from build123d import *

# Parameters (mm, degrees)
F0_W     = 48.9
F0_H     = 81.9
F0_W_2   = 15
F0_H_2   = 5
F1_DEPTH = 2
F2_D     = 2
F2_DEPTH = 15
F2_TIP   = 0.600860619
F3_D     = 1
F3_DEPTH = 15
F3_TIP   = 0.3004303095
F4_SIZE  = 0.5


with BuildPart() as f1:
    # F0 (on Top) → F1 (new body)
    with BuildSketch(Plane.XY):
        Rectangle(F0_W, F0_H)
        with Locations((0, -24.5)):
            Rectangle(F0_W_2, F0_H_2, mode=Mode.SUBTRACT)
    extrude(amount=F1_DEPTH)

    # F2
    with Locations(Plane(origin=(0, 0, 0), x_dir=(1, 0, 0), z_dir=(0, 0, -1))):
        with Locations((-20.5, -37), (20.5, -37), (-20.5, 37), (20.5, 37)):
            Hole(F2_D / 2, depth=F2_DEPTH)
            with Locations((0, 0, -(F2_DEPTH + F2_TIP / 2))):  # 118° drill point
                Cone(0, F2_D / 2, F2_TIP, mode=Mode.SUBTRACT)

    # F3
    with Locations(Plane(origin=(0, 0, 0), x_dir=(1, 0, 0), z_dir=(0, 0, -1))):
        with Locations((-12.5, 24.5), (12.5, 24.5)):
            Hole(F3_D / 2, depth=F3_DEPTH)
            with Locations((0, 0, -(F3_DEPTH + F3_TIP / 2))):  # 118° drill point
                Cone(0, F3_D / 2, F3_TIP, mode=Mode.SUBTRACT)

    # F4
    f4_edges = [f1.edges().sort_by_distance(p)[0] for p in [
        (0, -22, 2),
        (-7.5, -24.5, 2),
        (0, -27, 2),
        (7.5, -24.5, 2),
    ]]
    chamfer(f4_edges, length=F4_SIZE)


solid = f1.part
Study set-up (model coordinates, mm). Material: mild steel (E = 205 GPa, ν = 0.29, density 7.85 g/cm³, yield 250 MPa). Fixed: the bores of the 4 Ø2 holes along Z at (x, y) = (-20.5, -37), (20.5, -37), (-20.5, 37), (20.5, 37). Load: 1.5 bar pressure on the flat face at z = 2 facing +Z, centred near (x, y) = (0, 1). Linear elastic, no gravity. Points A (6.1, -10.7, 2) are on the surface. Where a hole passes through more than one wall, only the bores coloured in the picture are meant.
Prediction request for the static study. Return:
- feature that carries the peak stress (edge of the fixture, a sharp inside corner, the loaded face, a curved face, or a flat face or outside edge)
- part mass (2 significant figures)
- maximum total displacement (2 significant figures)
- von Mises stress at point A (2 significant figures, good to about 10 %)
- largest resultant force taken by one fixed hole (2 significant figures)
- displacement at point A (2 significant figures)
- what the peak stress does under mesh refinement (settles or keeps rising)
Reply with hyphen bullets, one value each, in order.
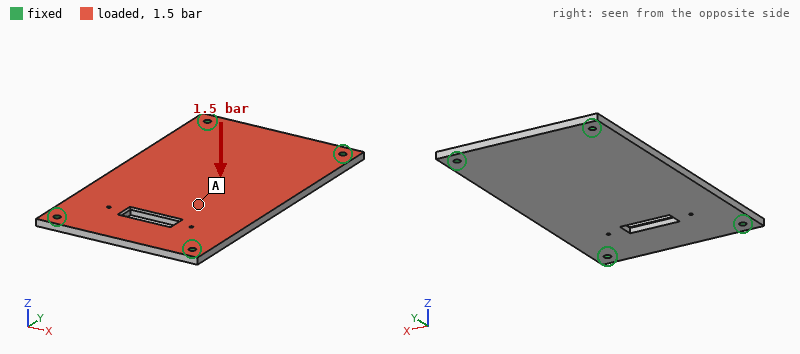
- edge of the fixture
- 61 g
- 0.13 mm
- 42 MPa
- 150 N
- 0.11 mm
- keeps rising
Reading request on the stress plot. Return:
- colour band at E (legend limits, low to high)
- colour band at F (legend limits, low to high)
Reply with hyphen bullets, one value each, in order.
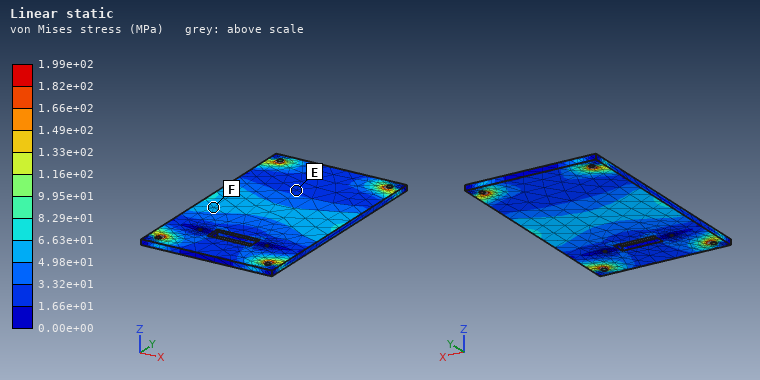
- 1.66e+01 to 3.32e+01 MPa
- 4.98e+01 to 6.63e+01 MPa
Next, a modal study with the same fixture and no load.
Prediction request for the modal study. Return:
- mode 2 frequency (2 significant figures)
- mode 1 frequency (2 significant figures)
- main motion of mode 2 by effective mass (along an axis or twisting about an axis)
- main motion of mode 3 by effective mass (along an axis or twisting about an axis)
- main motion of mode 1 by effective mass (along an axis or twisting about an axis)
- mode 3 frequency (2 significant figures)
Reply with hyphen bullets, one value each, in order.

- 2600 Hz
- 1600 Hz
- twisting about Y
- twisting about X
- along Z
- 4200 Hz
